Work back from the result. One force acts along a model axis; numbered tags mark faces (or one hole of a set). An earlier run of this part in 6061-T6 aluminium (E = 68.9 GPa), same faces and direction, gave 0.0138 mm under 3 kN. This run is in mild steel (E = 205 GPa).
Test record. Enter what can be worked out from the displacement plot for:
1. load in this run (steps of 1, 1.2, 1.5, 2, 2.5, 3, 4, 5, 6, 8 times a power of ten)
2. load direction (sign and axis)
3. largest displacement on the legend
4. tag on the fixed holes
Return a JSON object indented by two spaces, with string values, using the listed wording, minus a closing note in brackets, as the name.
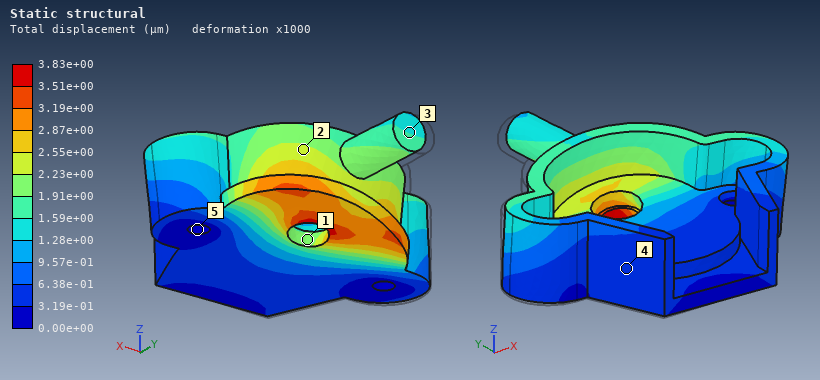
{
  "load in this run": "2.5 kN",
  "load direction": "+X",
  "largest displacement on the legend": "3.83e+00 µm",
  "tag on the fixed holes": "5"
}
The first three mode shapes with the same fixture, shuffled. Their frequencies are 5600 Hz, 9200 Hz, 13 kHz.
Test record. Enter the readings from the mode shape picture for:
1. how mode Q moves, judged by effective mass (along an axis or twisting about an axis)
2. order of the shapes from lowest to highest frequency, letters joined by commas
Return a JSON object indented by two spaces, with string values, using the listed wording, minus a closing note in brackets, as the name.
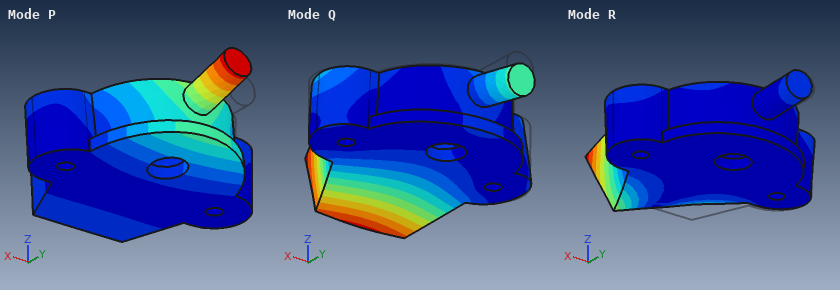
{
  "how mode Q moves, judged by effective mass": "along Z",
  "order of the shapes from lowest to highest frequency, letters joined by commas": "P, Q, R"
}
